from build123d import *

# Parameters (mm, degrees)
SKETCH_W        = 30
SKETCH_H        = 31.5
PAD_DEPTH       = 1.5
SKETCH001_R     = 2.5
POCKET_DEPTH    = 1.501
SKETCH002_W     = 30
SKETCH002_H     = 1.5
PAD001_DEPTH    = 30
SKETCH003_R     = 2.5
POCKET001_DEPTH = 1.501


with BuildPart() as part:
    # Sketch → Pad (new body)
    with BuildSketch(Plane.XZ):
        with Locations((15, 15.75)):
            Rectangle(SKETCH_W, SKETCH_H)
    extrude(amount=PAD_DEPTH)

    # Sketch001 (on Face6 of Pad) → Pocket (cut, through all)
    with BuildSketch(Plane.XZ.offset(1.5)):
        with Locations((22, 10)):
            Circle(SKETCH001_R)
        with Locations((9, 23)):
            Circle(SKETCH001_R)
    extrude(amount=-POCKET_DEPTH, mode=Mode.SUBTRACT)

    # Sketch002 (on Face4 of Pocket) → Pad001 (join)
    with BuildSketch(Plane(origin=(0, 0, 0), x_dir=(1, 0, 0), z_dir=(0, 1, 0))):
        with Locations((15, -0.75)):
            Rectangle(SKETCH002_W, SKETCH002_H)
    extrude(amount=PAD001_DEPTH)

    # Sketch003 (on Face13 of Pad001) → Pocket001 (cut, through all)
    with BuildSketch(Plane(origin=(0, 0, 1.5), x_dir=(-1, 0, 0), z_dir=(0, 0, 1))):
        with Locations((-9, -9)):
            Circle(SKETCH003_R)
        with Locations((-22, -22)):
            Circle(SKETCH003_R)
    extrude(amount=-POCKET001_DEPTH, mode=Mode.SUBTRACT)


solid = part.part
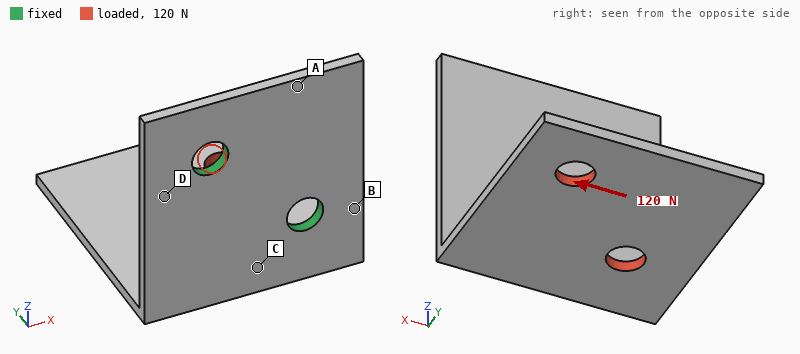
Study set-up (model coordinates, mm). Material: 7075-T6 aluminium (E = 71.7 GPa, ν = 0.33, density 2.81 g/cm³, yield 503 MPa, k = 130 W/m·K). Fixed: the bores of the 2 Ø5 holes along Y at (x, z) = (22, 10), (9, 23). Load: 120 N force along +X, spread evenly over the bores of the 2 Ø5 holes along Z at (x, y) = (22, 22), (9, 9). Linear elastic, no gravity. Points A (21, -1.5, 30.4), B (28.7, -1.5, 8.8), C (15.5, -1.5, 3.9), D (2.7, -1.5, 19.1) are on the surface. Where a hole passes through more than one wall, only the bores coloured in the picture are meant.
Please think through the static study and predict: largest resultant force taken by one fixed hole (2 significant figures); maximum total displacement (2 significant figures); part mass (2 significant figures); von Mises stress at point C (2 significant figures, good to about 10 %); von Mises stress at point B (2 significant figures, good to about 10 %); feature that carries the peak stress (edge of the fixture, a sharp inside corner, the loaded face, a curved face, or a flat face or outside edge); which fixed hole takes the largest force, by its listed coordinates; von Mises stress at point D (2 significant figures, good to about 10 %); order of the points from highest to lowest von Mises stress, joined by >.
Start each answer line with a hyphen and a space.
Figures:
- 140 N
- 0.53 mm
- 7.4 g
- 42 MPa
- 97 MPa
- a flat face or outside edge
- (22, 10)
- 68 MPa
- B > D > C > A
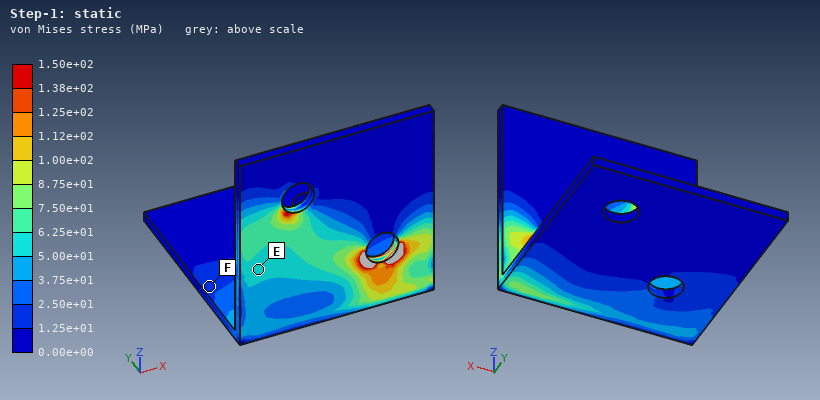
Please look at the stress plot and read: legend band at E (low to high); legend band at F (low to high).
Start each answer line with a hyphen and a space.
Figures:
- 5.00e+01 to 6.25e+01 MPa
- 1.25e+01 to 2.50e+01 MPa
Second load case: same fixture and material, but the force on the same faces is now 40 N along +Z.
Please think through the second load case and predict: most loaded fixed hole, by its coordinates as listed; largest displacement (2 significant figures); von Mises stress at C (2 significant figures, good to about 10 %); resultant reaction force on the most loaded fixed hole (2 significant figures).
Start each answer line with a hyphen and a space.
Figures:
- (22, 10)
- 0.53 mm
- 52 MPa
- 27 N
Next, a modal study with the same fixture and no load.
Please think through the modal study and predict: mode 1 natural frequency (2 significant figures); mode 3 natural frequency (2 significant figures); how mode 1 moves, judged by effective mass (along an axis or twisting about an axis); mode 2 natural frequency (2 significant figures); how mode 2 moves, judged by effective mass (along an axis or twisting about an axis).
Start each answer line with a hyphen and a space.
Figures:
- 890 Hz
- 2900 Hz
- along Z
- 1600 Hz
- along X
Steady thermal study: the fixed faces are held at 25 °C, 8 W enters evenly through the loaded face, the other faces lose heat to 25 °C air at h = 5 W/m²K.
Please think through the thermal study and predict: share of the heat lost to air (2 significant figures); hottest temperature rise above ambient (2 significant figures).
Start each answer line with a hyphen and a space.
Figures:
- 4.2 %
- 43 K
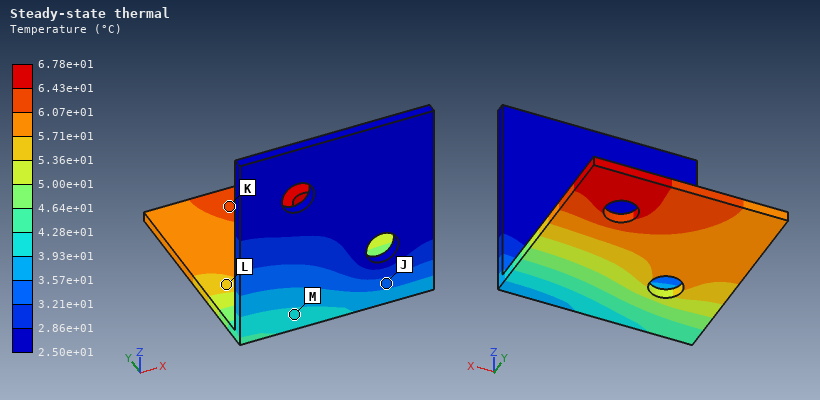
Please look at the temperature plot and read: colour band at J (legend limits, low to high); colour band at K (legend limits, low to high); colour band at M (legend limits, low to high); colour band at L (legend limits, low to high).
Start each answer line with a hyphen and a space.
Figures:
- 3.21e+01 to 3.57e+01 °C
- 6.07e+01 to 6.43e+01 °C
- 3.93e+01 to 4.28e+01 °C
- 5.36e+01 to 5.71e+01 °C
